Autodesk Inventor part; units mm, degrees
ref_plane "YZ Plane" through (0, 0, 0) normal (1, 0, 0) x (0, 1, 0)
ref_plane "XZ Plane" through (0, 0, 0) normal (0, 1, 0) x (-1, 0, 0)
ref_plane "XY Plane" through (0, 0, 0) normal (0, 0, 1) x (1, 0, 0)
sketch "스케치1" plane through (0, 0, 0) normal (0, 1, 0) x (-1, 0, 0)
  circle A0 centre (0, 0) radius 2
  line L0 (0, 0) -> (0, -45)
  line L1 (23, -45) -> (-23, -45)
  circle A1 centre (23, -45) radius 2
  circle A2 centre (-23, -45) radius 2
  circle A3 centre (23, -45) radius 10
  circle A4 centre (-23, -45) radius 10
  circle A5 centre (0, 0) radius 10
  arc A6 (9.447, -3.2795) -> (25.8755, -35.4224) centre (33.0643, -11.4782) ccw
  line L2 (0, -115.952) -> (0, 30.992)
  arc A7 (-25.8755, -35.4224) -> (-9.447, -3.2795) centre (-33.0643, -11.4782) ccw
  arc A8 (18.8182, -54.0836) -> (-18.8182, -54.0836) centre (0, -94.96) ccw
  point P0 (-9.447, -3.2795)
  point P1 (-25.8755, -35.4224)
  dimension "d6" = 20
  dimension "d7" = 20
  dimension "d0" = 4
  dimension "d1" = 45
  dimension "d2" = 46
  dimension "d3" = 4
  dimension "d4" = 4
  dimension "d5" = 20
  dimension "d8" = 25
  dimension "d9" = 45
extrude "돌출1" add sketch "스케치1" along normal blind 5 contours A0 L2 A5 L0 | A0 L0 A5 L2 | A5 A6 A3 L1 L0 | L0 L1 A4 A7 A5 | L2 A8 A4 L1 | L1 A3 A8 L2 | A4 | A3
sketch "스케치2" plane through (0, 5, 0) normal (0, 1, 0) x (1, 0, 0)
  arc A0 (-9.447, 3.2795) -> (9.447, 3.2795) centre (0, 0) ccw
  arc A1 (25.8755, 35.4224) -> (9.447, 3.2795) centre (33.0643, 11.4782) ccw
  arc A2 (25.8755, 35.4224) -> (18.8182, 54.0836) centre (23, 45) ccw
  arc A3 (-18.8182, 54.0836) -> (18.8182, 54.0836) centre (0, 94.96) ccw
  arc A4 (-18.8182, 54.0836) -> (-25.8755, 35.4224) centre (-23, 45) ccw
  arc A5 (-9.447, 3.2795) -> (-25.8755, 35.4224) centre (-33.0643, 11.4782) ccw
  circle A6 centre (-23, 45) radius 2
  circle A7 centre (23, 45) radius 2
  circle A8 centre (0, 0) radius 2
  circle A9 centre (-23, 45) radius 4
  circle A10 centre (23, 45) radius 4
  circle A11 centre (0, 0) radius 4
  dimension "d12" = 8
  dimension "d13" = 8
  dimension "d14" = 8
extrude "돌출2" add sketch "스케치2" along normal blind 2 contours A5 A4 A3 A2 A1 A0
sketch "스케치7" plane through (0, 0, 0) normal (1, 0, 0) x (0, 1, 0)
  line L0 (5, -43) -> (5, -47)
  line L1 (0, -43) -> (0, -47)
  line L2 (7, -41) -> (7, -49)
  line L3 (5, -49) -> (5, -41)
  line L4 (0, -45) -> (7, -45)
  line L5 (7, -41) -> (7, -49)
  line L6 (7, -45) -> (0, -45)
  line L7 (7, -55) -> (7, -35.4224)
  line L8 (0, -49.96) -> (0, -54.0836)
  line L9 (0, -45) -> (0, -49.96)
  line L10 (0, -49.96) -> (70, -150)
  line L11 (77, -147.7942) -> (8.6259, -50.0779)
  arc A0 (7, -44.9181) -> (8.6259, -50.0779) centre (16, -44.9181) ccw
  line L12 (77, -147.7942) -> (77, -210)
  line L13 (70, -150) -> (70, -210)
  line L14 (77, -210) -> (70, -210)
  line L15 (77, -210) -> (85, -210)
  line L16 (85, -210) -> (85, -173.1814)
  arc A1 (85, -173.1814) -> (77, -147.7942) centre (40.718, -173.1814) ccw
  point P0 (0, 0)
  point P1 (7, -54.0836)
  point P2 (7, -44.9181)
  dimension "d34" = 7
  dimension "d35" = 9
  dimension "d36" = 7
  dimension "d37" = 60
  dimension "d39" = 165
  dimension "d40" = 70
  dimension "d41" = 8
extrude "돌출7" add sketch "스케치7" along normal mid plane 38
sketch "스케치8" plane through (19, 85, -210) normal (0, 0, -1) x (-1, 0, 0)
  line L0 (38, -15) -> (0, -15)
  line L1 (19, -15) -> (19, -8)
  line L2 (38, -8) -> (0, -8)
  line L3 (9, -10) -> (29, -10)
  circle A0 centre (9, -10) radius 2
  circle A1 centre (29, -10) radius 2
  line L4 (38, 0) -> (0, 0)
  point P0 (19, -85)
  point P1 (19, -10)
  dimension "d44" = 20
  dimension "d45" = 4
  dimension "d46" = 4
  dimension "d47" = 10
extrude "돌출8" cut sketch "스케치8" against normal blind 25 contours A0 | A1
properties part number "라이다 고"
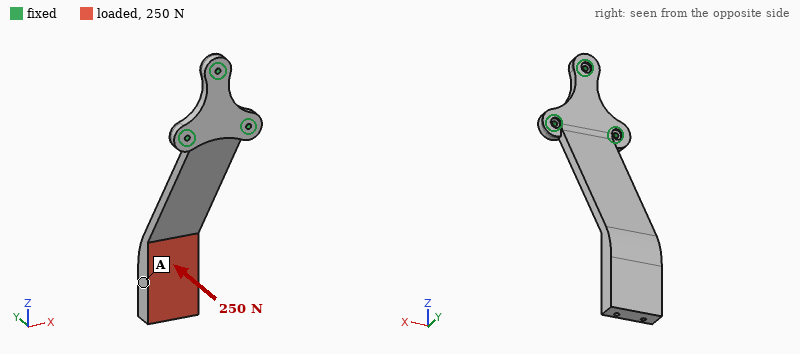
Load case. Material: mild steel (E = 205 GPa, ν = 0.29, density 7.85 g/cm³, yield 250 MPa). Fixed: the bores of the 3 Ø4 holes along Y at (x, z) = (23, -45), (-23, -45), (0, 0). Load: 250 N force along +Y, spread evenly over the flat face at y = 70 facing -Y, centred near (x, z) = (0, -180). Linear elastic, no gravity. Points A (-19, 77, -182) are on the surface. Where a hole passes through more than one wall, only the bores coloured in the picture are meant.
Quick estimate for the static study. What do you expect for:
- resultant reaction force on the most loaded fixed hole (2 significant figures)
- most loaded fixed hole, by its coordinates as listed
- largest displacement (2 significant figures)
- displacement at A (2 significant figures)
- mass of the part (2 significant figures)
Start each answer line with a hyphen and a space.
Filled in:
- 800 N
- (0, 0)
- 1.7 mm
- 1.3 mm
- 610 g
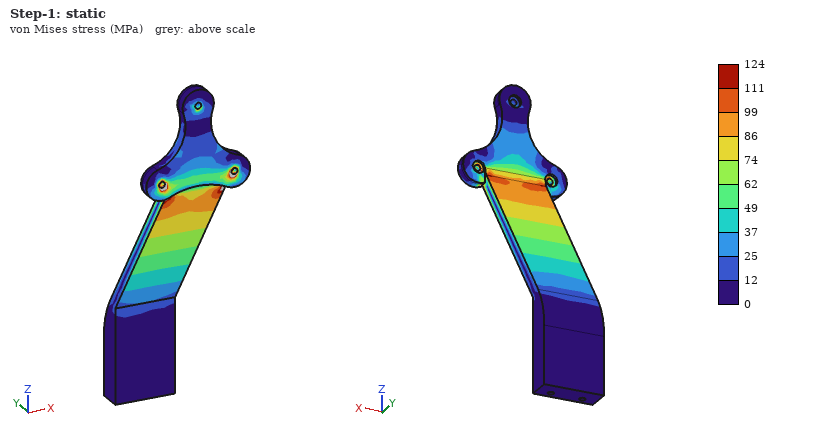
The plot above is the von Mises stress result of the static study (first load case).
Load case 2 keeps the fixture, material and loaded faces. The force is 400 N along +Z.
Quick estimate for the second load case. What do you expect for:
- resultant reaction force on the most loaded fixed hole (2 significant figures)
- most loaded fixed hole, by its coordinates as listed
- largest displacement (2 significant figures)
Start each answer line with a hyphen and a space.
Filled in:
- 720 N
- (0, 0)
- 1.1 mm
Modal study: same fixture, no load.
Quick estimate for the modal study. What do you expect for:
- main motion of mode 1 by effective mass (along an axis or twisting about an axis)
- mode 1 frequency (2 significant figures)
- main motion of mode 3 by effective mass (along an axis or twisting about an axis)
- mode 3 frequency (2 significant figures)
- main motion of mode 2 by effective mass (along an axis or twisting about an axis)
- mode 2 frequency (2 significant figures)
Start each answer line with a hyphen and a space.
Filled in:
- along Y
- 120 Hz
- along Z
- 880 Hz
- along X
- 540 Hz
